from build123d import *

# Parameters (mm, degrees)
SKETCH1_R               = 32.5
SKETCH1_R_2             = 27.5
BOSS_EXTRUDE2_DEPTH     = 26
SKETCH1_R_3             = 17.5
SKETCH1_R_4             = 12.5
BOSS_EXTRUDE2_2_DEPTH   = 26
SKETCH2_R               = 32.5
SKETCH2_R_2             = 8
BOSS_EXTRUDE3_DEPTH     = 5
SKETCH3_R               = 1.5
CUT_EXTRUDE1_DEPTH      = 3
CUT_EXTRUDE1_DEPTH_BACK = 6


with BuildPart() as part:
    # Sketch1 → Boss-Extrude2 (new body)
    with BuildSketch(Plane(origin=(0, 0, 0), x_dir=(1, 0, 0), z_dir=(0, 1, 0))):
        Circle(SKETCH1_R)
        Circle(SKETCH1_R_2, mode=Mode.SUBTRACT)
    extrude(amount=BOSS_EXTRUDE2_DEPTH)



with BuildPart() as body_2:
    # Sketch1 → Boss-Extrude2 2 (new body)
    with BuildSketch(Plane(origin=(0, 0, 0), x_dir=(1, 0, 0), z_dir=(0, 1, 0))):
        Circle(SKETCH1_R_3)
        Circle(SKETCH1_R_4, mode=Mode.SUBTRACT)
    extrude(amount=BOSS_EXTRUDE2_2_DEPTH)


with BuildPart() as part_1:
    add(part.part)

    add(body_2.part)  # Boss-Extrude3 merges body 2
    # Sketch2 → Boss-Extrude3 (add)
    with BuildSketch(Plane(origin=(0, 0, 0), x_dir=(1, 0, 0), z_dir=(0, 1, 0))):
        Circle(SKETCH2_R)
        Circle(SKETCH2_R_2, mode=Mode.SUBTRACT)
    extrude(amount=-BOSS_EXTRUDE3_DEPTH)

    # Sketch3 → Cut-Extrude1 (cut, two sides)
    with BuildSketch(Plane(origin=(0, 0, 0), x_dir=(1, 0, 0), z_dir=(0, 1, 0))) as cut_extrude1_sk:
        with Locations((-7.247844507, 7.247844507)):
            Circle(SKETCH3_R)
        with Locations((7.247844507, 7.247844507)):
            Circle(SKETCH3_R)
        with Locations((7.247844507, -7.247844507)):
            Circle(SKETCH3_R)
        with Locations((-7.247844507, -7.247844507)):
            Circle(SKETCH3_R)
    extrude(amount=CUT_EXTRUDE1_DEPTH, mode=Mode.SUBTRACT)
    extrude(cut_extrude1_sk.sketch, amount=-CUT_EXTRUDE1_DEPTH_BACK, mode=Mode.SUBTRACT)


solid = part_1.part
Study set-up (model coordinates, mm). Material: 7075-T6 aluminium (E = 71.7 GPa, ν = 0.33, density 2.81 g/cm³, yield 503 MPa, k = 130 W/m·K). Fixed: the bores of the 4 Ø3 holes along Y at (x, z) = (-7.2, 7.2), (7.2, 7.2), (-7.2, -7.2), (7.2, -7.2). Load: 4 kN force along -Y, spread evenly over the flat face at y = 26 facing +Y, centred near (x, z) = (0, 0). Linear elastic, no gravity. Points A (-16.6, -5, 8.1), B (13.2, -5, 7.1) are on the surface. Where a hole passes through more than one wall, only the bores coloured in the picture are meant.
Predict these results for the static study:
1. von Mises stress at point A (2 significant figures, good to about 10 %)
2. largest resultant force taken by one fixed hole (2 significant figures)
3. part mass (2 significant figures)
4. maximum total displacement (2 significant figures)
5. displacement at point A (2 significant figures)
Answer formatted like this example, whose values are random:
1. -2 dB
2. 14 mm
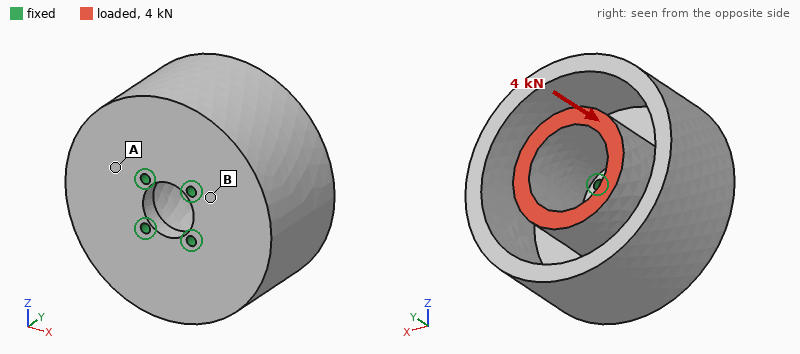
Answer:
1. 5.1 MPa
2. 1.0 kN
3. 150 g
4. 7.1 µm
5. 4.7 µm
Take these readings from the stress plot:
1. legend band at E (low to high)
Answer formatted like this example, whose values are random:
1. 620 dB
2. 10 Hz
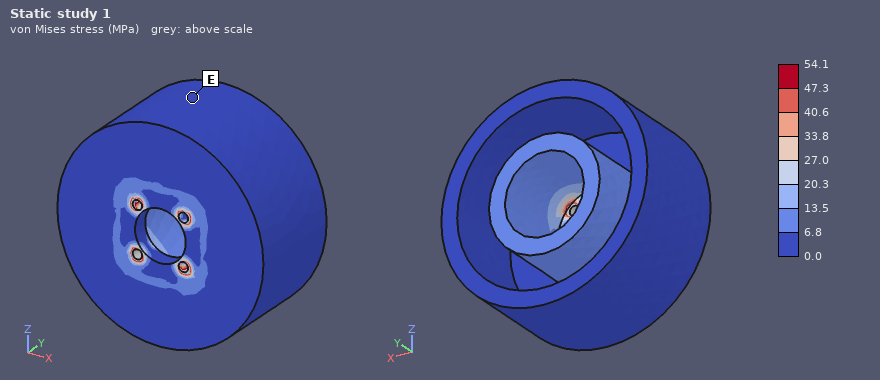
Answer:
1. 0.0 to 6.8 MPa
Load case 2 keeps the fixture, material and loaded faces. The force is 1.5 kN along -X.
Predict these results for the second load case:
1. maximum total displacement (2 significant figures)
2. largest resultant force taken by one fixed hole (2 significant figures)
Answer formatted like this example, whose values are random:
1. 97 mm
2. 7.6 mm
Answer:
1. 31 µm
2. 1.1 kN
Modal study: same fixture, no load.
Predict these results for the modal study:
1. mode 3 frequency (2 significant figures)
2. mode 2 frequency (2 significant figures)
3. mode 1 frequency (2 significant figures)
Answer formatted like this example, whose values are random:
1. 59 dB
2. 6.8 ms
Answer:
1. 5300 Hz
2. 3300 Hz
3. 3300 Hz
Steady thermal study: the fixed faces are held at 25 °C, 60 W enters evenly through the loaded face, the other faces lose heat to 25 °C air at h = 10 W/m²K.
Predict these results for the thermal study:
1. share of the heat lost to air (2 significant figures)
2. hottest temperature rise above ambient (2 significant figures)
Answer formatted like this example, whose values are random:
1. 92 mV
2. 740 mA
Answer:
1. 3.5 %
2. 33 K
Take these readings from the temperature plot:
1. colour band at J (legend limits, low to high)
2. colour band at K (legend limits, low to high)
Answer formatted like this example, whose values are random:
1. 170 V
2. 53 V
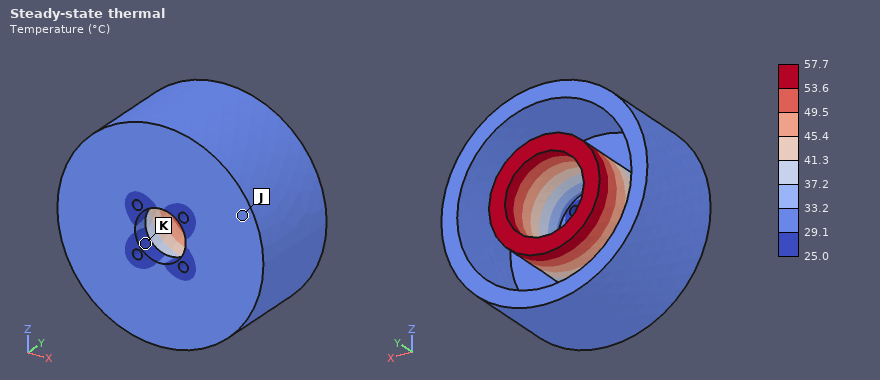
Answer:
1. 29.1 to 33.2 °C
2. 25.0 to 29.1 °C
